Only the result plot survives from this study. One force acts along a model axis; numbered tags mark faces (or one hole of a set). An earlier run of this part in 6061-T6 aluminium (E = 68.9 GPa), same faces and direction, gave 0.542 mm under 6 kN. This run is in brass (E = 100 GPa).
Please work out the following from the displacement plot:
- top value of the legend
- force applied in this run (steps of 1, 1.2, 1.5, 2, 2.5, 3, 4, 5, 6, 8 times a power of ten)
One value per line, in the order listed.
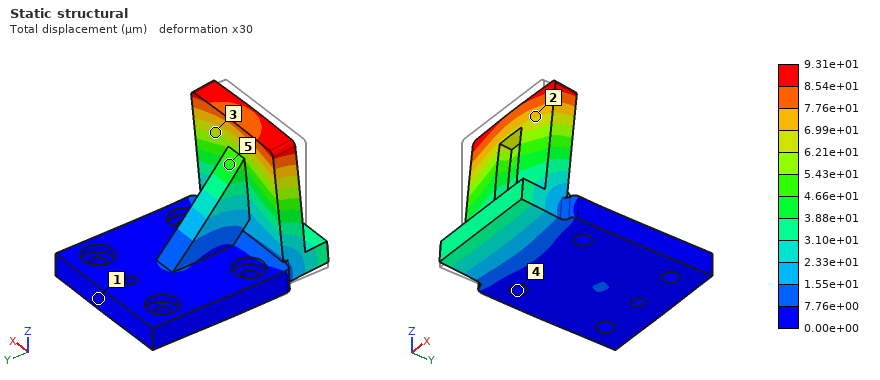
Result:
9.31e+01 µm
1.5 kN
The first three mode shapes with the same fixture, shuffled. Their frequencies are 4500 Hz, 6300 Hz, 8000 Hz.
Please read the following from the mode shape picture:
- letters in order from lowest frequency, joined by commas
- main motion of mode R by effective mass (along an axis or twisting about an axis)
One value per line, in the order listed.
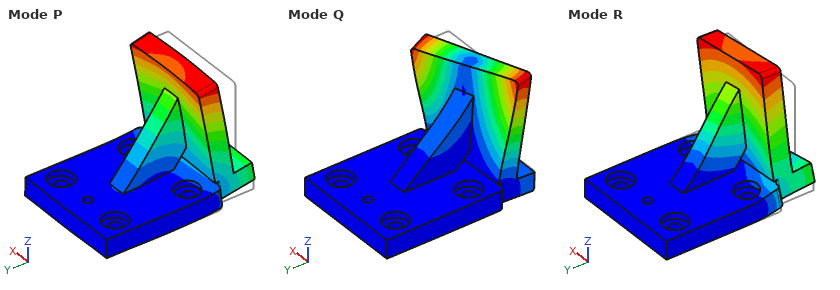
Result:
P, R, Q
along X
